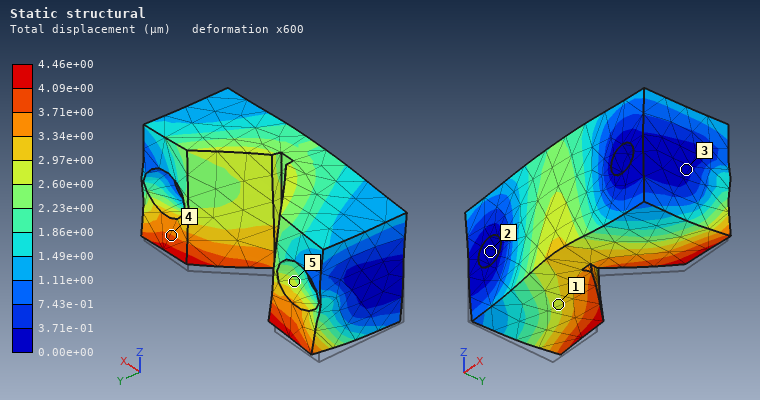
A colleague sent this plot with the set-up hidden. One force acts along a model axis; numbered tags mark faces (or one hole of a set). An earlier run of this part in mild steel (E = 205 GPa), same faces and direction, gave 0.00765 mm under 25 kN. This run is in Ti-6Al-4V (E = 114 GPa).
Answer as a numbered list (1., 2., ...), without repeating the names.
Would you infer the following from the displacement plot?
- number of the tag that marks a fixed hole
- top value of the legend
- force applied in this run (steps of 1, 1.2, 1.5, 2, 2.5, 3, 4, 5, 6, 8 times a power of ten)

1. 2
2. 4.46e+00 µm
3. 8 kN
